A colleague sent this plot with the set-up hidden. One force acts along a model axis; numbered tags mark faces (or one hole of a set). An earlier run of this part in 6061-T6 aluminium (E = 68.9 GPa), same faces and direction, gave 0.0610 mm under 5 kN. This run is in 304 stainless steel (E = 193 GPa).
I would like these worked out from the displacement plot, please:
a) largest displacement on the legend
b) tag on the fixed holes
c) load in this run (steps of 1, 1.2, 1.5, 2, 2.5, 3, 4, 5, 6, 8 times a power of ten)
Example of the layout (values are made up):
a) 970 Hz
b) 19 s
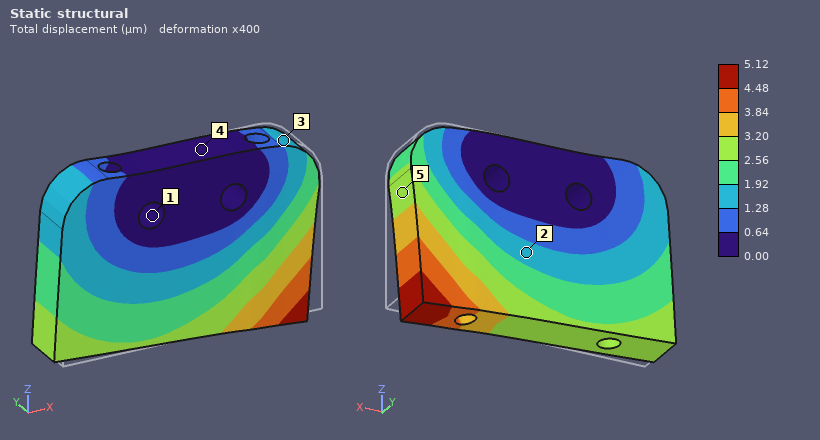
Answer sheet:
a) 5.12 µm
b) 1
c) 1.2 kN
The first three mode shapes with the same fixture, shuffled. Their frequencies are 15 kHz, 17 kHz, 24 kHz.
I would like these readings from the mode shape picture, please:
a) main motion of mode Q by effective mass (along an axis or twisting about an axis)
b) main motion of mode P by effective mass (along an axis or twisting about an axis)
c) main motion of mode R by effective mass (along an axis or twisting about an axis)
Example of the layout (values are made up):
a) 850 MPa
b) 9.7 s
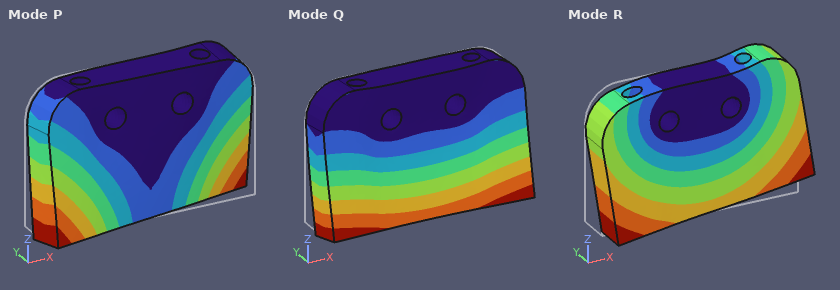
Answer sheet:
a) along Y
b) twisting about Z
c) along X
